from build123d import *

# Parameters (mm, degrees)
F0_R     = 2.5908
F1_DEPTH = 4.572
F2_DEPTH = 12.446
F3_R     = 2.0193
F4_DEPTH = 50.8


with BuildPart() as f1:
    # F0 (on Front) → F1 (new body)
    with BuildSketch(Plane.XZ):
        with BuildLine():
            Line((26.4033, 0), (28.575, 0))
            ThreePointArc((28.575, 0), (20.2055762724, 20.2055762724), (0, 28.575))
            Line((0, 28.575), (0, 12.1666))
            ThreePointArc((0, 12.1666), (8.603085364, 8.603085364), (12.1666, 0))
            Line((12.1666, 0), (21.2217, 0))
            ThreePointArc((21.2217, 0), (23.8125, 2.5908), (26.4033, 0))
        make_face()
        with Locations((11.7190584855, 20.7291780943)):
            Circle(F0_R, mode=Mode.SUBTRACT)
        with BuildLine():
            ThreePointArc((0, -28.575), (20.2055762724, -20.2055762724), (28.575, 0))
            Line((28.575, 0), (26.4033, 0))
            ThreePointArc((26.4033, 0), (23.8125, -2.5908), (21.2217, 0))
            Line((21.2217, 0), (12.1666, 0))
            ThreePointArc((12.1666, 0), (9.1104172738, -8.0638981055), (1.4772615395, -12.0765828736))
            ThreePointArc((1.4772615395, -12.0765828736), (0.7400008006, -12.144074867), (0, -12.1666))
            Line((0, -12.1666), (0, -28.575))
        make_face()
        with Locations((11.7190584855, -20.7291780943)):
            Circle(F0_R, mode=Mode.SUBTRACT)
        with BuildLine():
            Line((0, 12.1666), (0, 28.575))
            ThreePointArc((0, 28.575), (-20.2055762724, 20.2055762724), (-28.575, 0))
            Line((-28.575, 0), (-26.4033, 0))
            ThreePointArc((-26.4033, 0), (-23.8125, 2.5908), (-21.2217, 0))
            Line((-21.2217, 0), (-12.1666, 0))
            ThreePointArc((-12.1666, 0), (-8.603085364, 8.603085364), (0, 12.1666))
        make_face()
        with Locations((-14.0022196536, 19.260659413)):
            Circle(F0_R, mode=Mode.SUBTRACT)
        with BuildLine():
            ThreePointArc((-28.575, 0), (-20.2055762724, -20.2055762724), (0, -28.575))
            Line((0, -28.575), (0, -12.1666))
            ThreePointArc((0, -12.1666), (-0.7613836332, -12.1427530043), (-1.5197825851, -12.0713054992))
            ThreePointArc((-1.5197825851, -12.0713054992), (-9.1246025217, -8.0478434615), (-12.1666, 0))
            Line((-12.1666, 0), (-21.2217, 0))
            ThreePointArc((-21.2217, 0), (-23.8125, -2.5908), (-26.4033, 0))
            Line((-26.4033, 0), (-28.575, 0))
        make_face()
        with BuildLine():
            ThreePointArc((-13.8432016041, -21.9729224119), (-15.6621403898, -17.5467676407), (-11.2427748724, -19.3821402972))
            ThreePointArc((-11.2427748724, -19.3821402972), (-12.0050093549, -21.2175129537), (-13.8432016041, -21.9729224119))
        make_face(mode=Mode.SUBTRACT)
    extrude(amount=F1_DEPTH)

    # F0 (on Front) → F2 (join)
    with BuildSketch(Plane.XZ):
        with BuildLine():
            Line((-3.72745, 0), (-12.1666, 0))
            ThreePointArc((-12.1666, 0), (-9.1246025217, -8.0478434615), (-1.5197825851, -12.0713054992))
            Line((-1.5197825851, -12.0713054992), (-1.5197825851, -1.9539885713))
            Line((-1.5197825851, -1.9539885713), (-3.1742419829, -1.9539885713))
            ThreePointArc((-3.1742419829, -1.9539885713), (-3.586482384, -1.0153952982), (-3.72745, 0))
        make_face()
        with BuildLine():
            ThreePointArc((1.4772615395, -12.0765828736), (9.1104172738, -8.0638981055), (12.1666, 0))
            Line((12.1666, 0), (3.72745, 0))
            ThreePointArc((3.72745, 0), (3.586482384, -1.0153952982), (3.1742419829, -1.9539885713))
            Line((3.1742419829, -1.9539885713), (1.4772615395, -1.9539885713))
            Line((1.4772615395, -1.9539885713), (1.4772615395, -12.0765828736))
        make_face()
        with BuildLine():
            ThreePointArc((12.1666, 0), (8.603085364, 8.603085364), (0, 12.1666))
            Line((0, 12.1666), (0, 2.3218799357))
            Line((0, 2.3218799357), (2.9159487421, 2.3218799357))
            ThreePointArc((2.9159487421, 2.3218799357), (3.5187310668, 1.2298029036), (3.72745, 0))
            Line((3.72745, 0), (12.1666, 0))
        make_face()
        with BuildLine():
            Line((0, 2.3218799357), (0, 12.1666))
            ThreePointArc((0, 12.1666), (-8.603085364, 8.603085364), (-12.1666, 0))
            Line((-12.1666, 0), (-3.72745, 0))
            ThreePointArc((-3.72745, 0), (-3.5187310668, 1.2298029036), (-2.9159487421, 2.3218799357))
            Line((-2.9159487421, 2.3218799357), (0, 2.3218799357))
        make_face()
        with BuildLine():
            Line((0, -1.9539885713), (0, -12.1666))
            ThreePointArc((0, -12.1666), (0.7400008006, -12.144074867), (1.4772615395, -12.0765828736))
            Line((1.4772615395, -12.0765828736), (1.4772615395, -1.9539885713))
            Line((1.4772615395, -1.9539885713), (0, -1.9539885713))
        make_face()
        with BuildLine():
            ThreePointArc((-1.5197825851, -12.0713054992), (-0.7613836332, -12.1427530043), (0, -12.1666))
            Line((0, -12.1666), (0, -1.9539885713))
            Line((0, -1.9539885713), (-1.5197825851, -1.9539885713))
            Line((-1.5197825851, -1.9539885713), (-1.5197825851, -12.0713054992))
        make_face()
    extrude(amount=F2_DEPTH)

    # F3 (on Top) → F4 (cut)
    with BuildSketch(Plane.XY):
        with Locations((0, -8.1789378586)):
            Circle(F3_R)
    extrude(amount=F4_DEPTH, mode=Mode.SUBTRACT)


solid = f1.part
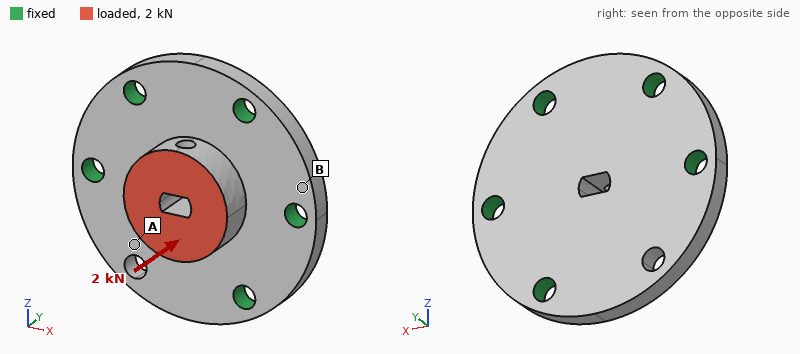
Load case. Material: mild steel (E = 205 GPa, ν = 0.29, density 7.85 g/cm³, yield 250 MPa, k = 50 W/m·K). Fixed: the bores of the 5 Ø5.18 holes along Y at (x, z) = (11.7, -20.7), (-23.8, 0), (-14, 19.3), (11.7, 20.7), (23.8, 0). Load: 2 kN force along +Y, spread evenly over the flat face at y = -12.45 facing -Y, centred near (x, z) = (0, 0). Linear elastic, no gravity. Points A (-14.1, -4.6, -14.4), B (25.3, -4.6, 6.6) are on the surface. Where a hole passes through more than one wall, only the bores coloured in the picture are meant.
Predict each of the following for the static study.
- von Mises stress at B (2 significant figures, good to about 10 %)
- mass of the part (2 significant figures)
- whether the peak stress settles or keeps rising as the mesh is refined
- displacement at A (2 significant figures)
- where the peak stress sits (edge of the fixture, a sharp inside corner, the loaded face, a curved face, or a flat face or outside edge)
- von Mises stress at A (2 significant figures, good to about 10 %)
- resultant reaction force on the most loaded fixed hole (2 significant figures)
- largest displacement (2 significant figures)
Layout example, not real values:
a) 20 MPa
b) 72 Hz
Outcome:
a) 6.9 MPa
b) 110 g
c) keeps rising
d) 3.8 µm
e) edge of the fixture
f) 14 MPa
g) 540 N
h) 5.2 µm
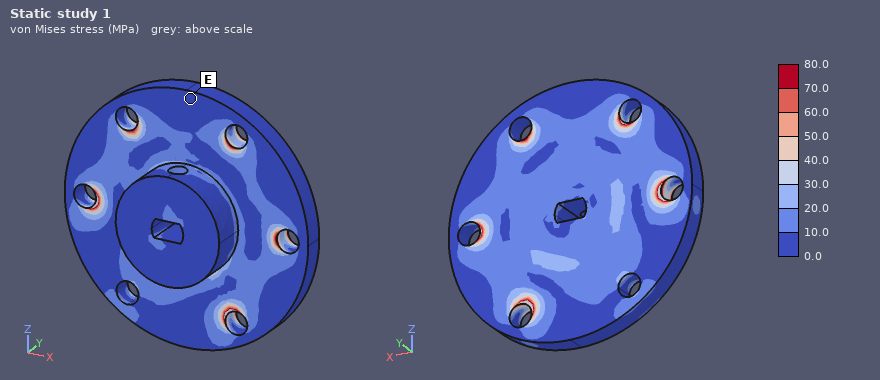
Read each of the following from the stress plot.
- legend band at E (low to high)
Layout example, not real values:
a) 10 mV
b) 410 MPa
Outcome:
a) 0.0 to 10.0 MPa
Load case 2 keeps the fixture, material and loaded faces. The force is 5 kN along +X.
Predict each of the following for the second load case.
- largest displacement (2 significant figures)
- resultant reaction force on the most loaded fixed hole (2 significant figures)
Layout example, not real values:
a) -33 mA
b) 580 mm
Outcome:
a) 12 µm
b) 1.8 kN
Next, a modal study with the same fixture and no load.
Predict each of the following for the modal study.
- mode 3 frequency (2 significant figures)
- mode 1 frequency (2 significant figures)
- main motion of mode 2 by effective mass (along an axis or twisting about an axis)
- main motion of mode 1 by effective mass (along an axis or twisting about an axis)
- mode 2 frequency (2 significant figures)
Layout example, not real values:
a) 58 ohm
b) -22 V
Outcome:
a) 24 kHz
b) 11 kHz
c) along Y
d) along Y
e) 17 kHz
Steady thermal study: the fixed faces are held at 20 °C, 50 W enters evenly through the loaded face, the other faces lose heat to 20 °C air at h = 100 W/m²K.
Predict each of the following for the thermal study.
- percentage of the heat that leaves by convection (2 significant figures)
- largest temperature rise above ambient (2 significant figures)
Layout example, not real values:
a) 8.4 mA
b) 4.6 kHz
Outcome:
a) 20 %
b) 54 K
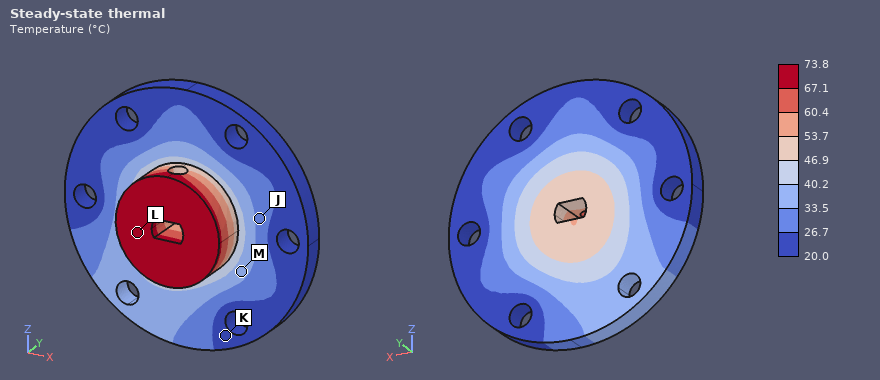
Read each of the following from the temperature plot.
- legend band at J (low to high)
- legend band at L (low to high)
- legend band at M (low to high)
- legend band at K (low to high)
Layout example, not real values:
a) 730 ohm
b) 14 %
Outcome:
a) 26.7 to 33.5 °C
b) 67.1 to 73.8 °C
c) 33.5 to 40.2 °C
d) 20.0 to 26.7 °C
